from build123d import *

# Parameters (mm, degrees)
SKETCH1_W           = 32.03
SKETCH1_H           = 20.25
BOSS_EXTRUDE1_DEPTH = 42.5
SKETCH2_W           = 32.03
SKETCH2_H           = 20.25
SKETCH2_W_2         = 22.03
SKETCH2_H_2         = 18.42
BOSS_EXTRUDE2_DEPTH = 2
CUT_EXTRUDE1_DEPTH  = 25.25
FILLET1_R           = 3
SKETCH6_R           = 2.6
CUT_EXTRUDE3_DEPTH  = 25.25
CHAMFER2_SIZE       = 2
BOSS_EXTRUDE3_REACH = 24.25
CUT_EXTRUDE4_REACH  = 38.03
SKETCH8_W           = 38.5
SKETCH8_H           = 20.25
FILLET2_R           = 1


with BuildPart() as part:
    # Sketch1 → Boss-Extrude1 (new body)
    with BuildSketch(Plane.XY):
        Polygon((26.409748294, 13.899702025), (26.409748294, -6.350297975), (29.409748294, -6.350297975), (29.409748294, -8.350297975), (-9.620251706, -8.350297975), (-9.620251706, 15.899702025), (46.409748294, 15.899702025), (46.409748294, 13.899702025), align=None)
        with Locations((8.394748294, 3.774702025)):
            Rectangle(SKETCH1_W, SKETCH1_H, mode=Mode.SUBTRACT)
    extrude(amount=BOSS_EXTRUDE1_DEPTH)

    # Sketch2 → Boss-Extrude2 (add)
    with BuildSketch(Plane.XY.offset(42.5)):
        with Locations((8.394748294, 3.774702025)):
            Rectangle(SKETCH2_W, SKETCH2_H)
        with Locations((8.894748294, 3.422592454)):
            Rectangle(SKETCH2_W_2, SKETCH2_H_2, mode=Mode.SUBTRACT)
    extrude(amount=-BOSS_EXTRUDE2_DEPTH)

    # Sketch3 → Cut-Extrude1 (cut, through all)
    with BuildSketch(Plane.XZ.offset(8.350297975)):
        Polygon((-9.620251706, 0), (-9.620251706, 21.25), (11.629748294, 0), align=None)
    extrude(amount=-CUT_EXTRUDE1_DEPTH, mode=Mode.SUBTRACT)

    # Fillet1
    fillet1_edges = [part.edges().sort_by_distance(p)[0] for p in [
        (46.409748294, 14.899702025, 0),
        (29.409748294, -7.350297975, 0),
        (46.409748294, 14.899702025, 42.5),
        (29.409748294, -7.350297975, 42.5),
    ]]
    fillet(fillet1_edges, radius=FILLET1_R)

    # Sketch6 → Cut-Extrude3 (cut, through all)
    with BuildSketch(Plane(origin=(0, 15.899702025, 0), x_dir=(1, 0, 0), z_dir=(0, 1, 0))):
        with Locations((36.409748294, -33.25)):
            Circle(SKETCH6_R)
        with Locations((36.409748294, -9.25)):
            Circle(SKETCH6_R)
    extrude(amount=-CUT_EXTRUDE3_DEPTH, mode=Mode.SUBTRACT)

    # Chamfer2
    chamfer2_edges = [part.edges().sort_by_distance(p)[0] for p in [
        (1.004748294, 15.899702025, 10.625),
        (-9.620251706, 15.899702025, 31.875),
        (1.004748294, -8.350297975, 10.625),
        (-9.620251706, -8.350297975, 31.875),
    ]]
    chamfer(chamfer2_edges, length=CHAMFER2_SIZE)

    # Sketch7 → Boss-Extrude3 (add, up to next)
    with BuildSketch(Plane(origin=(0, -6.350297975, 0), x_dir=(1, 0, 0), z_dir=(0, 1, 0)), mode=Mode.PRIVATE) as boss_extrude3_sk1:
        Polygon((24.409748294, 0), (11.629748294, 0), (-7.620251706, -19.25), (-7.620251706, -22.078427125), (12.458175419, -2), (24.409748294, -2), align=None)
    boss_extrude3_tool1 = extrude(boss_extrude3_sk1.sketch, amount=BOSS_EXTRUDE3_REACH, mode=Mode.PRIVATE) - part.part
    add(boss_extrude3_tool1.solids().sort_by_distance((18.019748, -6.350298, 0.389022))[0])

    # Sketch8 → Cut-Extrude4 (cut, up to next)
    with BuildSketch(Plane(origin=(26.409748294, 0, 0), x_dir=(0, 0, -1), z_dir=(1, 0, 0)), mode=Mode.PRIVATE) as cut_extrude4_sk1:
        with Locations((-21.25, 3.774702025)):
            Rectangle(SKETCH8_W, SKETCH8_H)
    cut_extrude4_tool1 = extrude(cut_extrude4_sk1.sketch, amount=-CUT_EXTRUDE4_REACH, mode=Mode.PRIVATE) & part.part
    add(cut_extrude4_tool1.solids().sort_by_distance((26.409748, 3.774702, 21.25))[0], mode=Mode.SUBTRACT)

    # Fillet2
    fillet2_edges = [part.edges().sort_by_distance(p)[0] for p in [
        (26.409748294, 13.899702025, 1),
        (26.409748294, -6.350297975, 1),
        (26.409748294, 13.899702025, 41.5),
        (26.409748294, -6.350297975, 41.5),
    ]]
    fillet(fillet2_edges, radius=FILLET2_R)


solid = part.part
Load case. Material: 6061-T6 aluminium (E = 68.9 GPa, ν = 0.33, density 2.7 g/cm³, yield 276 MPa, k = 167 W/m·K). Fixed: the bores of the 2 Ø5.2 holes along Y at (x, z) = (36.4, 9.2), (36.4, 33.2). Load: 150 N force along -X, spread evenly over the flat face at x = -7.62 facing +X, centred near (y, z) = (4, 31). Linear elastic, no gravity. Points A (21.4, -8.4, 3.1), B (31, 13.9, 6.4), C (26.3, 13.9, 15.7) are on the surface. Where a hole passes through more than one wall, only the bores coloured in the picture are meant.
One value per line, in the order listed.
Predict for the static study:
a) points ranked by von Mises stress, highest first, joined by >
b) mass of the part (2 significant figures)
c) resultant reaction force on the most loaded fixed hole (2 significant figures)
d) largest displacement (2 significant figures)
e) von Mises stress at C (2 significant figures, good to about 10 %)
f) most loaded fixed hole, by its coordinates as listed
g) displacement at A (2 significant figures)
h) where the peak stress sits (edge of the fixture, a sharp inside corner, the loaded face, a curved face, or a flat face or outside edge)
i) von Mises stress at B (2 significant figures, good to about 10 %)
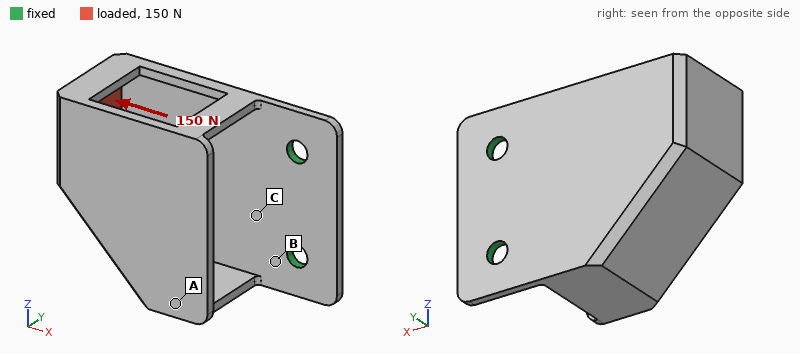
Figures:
B > C > A
27 g
130 N
0.49 mm
37 MPa
(36.4, 33.2)
0.26 mm
a curved face
64 MPa
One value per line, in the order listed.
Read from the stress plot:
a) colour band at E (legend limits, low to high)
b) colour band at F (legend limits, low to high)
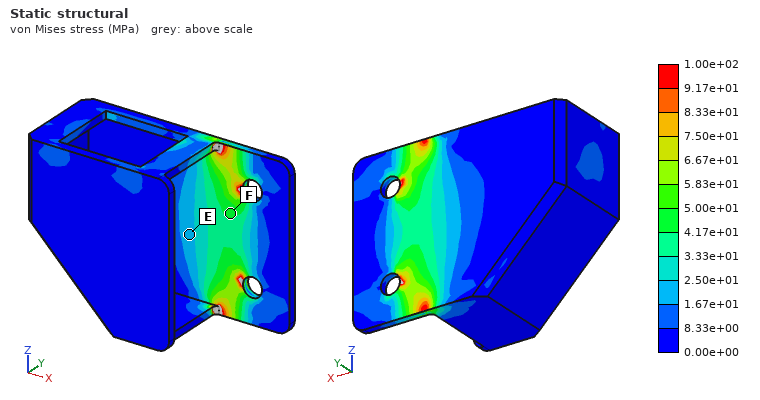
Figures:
1.67e+01 to 2.50e+01 MPa
4.17e+01 to 5.00e+01 MPa
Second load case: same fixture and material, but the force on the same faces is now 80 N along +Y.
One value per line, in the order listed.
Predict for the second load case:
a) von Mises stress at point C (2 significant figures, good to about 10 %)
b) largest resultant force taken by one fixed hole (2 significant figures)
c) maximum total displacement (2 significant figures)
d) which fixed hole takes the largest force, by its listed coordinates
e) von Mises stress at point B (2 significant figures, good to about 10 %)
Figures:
66 MPa
66 N
0.87 mm
(36.4, 33.2)
110 MPa
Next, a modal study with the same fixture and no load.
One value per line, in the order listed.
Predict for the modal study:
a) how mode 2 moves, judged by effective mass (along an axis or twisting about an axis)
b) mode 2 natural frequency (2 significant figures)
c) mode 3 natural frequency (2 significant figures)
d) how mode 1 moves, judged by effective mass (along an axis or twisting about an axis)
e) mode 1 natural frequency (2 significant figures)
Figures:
along Z
1200 Hz
2900 Hz
along Y
470 Hz
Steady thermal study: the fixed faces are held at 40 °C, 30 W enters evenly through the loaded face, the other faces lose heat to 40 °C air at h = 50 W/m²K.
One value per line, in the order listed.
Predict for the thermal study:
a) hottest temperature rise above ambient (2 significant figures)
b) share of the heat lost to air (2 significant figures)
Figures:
59 K
48 %
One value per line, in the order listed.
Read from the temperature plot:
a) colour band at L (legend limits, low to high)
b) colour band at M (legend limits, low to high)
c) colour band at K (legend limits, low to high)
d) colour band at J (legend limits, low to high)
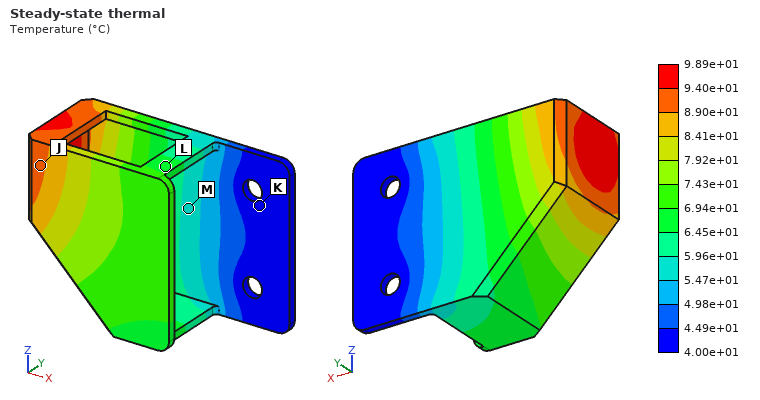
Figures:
6.45e+01 to 6.94e+01 °C
5.47e+01 to 5.96e+01 °C
4.00e+01 to 4.49e+01 °C
8.90e+01 to 9.40e+01 °C
